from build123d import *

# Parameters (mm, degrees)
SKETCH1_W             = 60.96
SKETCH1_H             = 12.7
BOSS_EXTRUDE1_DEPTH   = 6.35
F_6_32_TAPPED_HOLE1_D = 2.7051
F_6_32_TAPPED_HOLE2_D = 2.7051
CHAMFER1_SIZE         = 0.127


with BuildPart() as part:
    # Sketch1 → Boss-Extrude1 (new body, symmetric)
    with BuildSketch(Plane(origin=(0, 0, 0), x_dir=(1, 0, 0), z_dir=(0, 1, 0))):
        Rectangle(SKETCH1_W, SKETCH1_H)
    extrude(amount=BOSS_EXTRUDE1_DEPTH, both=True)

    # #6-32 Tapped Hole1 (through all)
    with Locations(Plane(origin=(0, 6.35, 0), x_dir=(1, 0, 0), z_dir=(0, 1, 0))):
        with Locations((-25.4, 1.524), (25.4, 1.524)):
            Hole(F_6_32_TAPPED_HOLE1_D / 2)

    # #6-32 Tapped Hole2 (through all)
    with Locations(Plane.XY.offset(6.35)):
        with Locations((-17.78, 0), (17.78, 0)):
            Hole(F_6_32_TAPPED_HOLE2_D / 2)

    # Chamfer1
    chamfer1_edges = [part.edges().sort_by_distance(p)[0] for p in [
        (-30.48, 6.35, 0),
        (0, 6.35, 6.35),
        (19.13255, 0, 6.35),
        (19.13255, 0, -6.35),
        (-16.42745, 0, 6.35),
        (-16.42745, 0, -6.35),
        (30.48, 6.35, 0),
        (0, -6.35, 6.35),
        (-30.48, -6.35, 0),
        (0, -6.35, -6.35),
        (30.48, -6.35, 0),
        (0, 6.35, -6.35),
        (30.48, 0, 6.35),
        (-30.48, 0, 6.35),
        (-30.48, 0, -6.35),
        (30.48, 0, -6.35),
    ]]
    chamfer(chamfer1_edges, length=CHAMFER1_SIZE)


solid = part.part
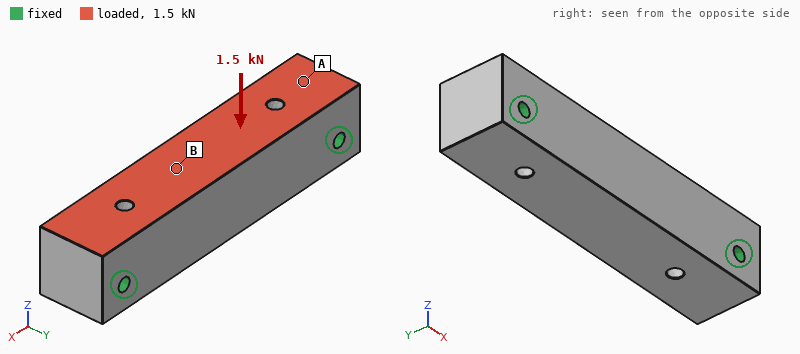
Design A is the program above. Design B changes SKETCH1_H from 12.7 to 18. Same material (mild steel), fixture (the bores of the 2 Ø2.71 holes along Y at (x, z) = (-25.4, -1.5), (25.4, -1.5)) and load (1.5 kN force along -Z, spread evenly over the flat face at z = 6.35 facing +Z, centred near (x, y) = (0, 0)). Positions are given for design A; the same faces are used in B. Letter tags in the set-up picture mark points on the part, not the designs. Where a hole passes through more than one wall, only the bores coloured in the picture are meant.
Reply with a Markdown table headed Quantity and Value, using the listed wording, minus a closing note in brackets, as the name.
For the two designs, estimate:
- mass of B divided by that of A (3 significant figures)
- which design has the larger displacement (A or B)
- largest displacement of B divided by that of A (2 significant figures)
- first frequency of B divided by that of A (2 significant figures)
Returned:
| Quantity | Value |
|---|---|
| mass of B divided by that of A | 1.42 |
| which design has the larger displacement | A |
| largest displacement of B divided by that of A | 0.56 |
| first frequency of B divided by that of A | 1.1 |
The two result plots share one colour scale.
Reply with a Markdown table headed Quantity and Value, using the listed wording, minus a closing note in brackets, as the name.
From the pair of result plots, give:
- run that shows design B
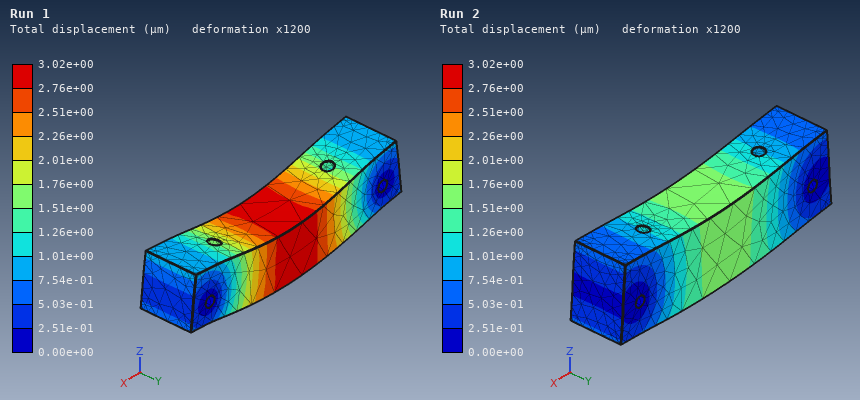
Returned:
| Quantity | Value |
|---|---|
| run that shows design B | Run 2 |
